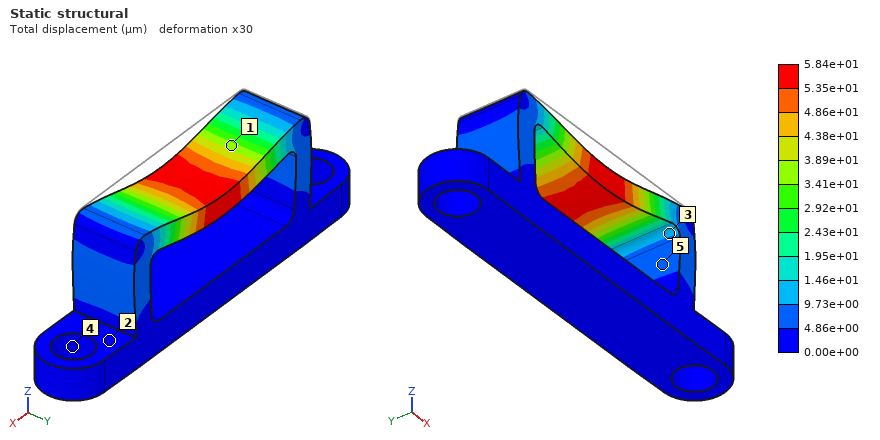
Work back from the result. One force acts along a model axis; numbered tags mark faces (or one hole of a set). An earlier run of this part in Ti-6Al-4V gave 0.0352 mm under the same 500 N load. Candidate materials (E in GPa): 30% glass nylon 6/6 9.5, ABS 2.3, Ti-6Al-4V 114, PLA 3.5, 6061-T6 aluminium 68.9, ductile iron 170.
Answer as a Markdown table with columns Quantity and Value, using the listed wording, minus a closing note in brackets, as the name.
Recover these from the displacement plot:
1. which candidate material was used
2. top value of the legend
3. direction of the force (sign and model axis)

| Quantity | Value |
|---|---|
| which candidate material was used | 6061-T6 aluminium |
| top value of the legend | 5.84e+01 µm |
| direction of the force | -Z |
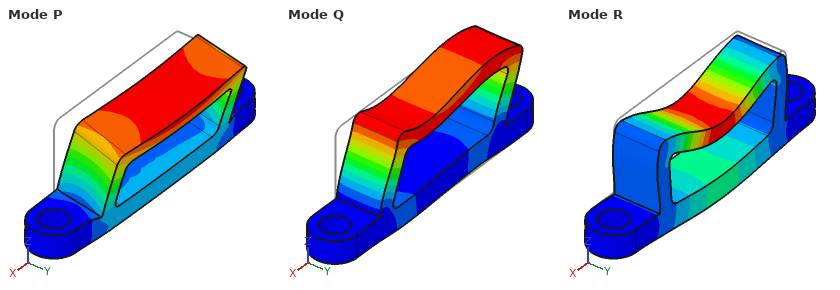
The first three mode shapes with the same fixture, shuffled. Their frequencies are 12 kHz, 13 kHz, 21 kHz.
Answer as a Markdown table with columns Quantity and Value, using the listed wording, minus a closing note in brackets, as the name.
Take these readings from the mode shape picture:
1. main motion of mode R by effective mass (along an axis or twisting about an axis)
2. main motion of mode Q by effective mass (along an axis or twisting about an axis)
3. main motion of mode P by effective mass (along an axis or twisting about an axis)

| Quantity | Value |
|---|---|
| main motion of mode R by effective mass | along Z |
| main motion of mode Q by effective mass | along X |
| main motion of mode P by effective mass | along Y |
